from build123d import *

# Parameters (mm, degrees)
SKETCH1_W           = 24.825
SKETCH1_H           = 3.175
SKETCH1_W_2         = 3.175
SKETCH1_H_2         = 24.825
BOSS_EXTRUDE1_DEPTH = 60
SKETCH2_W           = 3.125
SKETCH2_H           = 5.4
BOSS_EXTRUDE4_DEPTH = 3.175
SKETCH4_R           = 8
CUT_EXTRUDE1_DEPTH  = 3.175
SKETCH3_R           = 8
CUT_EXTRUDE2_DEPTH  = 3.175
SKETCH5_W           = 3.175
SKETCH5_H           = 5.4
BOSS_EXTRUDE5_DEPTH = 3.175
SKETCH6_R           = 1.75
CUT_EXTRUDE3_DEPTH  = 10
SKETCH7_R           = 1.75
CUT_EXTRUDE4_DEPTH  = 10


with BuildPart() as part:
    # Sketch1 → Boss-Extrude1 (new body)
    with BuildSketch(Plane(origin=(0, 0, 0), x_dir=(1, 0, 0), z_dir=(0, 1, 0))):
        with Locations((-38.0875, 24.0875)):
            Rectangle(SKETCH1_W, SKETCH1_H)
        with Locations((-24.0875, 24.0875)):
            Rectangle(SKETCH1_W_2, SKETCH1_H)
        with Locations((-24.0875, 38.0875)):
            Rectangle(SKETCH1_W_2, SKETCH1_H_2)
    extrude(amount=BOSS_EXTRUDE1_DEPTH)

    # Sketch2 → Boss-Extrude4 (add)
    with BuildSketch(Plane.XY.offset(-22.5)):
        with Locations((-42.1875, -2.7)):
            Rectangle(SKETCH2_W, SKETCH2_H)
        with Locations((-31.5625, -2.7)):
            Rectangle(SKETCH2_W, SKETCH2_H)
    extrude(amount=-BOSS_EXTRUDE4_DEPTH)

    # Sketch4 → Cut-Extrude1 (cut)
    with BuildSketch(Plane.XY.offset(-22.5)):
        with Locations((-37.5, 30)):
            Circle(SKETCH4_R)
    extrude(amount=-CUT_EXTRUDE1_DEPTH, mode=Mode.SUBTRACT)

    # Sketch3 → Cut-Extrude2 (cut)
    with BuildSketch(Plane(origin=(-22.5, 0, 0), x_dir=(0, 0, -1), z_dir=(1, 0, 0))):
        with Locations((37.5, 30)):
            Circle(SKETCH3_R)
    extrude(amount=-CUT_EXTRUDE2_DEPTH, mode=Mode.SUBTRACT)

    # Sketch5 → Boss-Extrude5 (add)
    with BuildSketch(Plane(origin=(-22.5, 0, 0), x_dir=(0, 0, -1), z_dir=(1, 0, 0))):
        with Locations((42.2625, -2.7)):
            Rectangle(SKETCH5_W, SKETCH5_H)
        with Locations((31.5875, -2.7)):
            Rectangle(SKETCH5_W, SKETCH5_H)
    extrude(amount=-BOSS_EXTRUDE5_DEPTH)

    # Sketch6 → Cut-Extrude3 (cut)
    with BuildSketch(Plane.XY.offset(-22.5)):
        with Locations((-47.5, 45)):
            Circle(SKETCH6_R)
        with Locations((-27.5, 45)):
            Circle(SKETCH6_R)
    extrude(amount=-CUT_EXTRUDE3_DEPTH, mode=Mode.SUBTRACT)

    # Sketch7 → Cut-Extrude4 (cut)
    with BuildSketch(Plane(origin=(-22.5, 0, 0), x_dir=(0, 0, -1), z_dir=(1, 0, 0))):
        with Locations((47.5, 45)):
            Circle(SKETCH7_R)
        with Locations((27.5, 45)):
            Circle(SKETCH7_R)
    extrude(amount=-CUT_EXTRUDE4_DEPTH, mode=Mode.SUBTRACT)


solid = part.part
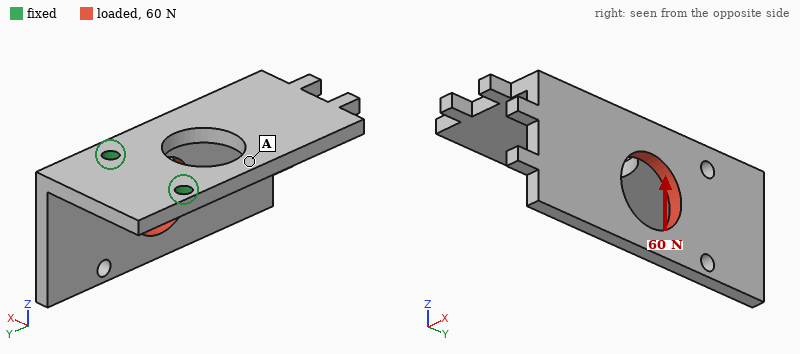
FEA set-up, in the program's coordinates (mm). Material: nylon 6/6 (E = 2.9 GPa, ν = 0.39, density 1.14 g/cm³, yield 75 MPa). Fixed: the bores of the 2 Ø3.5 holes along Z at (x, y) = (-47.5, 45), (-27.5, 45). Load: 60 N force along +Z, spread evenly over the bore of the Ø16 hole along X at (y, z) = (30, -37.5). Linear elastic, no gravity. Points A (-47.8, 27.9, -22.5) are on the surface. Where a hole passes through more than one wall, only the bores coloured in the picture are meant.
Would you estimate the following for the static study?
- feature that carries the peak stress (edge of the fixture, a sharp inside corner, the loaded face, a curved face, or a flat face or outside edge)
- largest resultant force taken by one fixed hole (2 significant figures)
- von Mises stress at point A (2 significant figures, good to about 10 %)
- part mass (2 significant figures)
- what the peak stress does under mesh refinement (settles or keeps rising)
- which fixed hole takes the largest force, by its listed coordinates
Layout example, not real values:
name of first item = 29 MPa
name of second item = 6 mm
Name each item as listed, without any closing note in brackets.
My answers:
feature that carries the peak stress = edge of the fixture
largest resultant force taken by one fixed hole = 62 N
von Mises stress at point A = 2.8 MPa
part mass = 10 g
what the peak stress does under mesh refinement = keeps rising
which fixed hole takes the largest force, by its listed coordinates = (-27.5, 45)
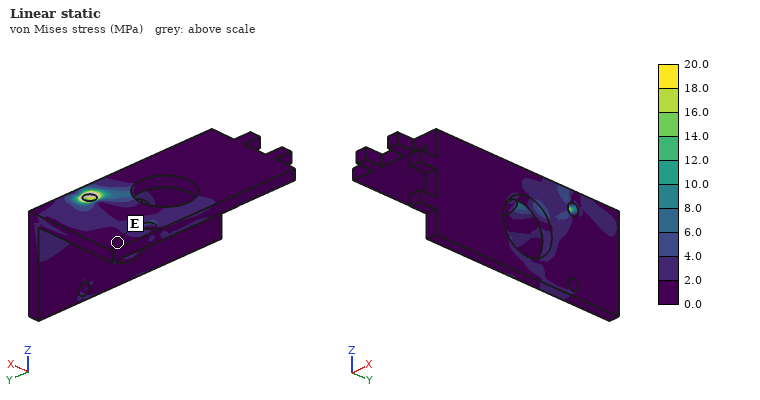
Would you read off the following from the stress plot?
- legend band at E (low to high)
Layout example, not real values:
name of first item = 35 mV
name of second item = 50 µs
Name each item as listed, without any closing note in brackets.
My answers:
legend band at E = 0.0 to 2.0 MPa
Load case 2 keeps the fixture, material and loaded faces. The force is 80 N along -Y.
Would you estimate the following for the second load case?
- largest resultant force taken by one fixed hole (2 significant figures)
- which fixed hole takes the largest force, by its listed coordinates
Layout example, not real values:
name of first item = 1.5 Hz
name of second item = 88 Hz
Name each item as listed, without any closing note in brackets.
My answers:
largest resultant force taken by one fixed hole = 88 N
which fixed hole takes the largest force, by its listed coordinates = (-27.5, 45)
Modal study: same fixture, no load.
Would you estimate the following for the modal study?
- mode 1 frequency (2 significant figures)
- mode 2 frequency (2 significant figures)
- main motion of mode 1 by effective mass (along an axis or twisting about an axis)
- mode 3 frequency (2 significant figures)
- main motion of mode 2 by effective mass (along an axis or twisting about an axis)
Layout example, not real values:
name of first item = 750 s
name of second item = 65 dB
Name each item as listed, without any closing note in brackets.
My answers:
mode 1 frequency = 500 Hz
mode 2 frequency = 610 Hz
main motion of mode 1 by effective mass = along Z
mode 3 frequency = 1100 Hz
main motion of mode 2 by effective mass = along X
